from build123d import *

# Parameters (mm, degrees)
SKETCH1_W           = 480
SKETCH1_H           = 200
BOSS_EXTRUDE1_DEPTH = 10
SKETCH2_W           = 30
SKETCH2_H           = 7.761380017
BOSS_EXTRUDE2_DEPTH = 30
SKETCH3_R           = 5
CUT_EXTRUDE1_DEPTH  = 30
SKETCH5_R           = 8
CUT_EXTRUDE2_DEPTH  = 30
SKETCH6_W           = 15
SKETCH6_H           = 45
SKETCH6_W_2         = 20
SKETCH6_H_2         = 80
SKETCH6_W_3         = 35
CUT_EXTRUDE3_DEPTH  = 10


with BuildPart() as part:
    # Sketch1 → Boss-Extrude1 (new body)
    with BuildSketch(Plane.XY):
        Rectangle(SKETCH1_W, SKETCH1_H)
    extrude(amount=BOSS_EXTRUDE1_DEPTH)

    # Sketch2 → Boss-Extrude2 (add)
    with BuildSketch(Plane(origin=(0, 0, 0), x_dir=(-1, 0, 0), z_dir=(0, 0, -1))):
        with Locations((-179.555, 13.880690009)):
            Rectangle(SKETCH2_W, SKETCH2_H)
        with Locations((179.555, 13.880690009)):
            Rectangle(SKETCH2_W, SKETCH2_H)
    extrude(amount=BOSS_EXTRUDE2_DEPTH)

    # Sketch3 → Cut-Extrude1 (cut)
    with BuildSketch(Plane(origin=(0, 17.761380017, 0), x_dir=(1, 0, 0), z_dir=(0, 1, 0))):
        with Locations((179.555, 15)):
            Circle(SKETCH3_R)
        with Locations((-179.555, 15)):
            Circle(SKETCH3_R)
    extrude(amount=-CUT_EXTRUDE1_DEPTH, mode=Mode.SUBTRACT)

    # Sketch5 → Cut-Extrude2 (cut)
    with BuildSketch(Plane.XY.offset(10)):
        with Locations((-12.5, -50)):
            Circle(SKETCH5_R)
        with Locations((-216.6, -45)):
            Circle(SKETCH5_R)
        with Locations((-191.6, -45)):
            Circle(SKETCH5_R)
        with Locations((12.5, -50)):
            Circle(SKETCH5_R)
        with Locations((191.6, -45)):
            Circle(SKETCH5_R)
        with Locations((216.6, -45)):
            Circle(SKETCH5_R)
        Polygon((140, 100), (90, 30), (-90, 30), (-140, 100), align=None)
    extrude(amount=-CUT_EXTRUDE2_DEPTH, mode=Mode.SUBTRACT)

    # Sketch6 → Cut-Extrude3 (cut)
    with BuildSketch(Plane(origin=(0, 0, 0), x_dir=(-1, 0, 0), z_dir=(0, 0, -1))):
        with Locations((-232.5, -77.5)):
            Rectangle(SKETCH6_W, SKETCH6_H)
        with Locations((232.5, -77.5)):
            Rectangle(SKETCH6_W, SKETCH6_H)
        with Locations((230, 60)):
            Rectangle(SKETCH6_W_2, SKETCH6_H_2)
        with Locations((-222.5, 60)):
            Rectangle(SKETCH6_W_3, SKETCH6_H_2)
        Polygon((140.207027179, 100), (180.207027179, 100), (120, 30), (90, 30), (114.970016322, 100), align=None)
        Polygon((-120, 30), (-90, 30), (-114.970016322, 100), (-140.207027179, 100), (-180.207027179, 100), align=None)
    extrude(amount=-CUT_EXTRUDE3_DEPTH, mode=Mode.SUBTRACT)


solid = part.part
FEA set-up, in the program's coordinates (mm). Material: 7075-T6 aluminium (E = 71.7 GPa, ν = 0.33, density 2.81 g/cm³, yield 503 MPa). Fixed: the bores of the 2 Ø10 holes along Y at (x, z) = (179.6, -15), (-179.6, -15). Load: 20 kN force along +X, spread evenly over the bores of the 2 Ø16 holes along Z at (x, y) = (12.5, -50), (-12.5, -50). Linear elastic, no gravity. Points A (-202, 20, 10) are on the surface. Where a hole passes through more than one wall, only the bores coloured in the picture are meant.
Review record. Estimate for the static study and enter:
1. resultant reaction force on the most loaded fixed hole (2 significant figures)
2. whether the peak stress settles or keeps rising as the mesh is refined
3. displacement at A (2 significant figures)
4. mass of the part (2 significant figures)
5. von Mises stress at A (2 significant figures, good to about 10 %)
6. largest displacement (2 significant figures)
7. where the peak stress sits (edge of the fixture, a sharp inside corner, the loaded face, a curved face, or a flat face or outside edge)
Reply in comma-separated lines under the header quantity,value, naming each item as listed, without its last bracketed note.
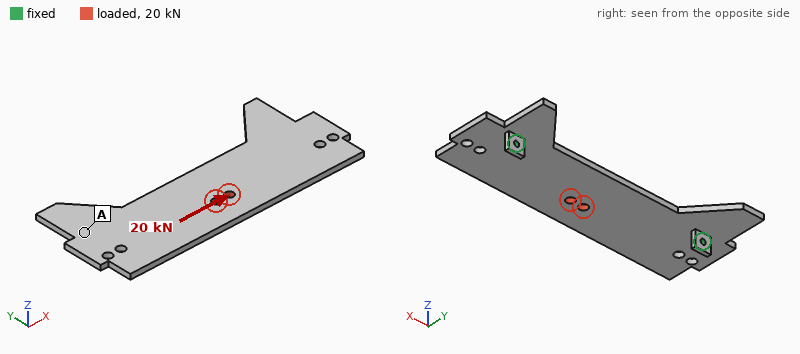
quantity,value
resultant reaction force on the most loaded fixed hole,11 kN
whether the peak stress settles or keeps rising as the mesh is refined,keeps rising
displacement at A,0.14 mm
mass of the part,1.9 kg
von Mises stress at A,12 MPa
largest displacement,0.36 mm
where the peak stress sits,edge of the fixture
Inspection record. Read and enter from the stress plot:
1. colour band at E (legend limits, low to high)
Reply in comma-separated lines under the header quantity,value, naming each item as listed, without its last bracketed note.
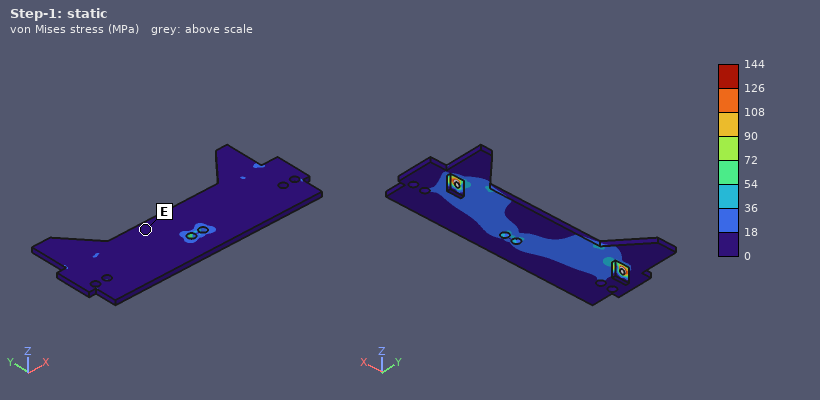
quantity,value
colour band at E,0 to 18 MPa
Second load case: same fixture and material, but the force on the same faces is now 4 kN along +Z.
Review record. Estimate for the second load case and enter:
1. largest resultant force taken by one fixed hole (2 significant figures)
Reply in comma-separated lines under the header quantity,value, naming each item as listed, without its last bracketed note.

quantity,value
largest resultant force taken by one fixed hole,5.1 kN
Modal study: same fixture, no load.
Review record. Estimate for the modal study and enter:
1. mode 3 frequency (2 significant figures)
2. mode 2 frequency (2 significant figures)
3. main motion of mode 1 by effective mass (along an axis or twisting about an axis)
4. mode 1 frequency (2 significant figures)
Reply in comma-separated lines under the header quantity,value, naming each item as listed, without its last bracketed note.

quantity,value
mode 3 frequency,430 Hz
mode 2 frequency,380 Hz
main motion of mode 1 by effective mass,along Z
mode 1 frequency,180 Hz
